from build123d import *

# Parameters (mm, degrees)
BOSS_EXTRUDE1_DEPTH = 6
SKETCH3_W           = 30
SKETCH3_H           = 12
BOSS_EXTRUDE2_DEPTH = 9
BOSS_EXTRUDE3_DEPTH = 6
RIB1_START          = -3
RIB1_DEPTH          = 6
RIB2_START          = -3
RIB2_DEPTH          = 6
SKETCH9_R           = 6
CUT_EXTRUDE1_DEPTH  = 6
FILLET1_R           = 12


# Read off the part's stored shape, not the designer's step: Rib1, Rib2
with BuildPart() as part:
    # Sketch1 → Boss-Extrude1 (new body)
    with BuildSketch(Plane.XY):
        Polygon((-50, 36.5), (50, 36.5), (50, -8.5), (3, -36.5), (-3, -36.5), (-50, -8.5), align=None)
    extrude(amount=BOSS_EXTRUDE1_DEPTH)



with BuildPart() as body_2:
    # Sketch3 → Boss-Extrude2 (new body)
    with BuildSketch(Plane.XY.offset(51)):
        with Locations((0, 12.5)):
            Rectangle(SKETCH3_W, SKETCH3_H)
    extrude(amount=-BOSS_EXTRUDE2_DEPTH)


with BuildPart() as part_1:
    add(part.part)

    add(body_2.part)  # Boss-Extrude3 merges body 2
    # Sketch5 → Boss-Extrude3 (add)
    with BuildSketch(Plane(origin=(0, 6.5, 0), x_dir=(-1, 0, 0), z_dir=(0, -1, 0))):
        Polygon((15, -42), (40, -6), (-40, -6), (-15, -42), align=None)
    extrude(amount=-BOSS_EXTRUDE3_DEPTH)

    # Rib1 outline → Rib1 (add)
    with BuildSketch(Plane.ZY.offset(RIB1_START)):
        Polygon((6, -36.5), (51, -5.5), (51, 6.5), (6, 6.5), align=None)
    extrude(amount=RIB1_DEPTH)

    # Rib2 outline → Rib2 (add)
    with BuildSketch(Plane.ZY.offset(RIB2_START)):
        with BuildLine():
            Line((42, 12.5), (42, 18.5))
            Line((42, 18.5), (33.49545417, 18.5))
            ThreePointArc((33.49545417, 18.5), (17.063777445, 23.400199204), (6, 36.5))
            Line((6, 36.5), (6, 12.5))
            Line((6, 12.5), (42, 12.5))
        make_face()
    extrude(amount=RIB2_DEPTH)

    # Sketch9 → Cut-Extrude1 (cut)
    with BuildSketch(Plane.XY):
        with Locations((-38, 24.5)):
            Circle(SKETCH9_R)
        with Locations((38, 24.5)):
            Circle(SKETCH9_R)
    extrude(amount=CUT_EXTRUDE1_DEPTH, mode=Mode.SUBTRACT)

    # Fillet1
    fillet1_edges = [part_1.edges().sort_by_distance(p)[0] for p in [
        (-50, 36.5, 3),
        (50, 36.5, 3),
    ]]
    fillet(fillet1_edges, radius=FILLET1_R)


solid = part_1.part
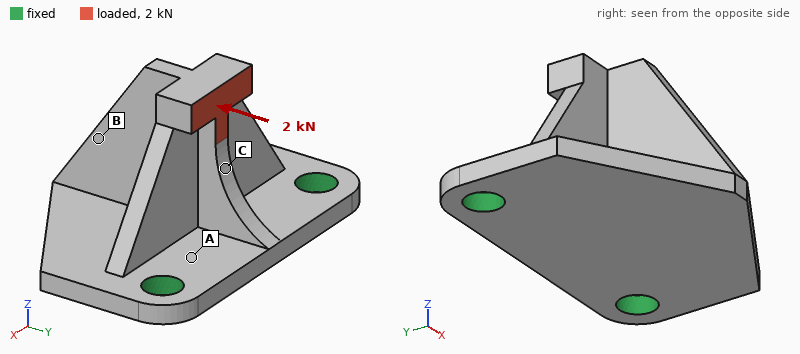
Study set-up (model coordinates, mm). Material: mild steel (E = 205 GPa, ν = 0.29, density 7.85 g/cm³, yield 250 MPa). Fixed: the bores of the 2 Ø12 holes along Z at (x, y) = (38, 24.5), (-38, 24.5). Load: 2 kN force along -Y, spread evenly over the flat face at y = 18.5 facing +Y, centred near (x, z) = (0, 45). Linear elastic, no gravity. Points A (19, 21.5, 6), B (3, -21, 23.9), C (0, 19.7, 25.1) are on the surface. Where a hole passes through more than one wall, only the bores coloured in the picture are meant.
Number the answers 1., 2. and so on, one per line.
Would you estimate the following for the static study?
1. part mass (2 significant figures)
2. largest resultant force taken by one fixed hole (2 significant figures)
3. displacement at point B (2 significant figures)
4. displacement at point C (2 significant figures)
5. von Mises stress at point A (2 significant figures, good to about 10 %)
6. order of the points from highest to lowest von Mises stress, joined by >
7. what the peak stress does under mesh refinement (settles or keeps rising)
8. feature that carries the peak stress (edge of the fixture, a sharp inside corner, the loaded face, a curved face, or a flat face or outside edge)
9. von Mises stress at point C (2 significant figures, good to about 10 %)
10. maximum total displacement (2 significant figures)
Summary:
1. 460 g
2. 1.0 kN
3. 0.15 mm
4. 0.081 mm
5. 96 MPa
6. A > C > B
7. keeps rising
8. edge of the fixture
9. 58 MPa
10. 0.19 mm
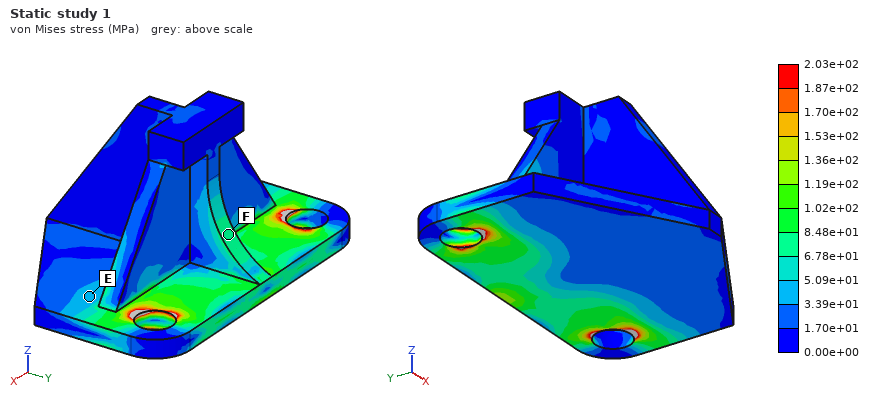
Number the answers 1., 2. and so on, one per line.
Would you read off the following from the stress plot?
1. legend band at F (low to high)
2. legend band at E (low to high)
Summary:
1. 6.78e+01 to 8.48e+01 MPa
2. 3.39e+01 to 5.09e+01 MPa
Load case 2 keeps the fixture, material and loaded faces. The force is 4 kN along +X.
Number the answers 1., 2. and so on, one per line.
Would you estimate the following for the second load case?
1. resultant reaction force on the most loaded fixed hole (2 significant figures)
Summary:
1. 3.1 kN
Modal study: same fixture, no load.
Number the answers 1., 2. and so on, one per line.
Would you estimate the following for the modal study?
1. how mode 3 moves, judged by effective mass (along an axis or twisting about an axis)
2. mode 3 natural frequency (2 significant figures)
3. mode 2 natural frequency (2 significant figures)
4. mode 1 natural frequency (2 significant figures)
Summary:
1. along Z
2. 5400 Hz
3. 5000 Hz
4. 1500 Hz
